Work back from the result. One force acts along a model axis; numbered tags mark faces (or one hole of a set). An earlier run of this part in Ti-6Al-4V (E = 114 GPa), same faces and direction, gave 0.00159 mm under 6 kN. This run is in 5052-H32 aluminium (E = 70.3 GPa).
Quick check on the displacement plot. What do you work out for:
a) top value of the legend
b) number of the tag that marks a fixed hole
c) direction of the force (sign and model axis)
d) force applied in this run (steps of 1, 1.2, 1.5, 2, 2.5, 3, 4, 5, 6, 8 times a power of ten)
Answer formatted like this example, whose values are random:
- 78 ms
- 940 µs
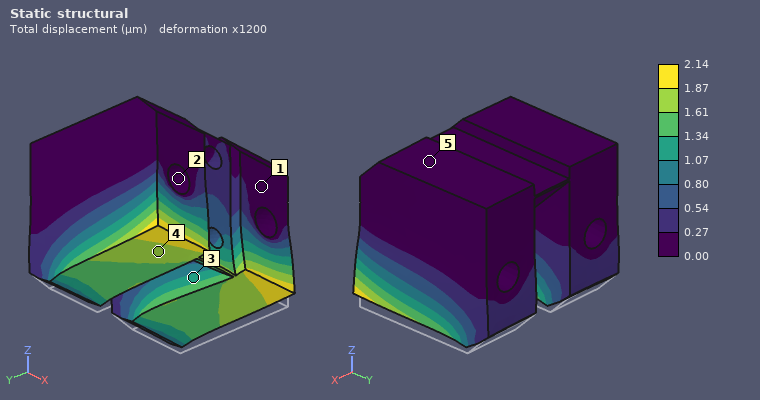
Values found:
- 2.14 µm
- 2
- +Z
- 5 kN
